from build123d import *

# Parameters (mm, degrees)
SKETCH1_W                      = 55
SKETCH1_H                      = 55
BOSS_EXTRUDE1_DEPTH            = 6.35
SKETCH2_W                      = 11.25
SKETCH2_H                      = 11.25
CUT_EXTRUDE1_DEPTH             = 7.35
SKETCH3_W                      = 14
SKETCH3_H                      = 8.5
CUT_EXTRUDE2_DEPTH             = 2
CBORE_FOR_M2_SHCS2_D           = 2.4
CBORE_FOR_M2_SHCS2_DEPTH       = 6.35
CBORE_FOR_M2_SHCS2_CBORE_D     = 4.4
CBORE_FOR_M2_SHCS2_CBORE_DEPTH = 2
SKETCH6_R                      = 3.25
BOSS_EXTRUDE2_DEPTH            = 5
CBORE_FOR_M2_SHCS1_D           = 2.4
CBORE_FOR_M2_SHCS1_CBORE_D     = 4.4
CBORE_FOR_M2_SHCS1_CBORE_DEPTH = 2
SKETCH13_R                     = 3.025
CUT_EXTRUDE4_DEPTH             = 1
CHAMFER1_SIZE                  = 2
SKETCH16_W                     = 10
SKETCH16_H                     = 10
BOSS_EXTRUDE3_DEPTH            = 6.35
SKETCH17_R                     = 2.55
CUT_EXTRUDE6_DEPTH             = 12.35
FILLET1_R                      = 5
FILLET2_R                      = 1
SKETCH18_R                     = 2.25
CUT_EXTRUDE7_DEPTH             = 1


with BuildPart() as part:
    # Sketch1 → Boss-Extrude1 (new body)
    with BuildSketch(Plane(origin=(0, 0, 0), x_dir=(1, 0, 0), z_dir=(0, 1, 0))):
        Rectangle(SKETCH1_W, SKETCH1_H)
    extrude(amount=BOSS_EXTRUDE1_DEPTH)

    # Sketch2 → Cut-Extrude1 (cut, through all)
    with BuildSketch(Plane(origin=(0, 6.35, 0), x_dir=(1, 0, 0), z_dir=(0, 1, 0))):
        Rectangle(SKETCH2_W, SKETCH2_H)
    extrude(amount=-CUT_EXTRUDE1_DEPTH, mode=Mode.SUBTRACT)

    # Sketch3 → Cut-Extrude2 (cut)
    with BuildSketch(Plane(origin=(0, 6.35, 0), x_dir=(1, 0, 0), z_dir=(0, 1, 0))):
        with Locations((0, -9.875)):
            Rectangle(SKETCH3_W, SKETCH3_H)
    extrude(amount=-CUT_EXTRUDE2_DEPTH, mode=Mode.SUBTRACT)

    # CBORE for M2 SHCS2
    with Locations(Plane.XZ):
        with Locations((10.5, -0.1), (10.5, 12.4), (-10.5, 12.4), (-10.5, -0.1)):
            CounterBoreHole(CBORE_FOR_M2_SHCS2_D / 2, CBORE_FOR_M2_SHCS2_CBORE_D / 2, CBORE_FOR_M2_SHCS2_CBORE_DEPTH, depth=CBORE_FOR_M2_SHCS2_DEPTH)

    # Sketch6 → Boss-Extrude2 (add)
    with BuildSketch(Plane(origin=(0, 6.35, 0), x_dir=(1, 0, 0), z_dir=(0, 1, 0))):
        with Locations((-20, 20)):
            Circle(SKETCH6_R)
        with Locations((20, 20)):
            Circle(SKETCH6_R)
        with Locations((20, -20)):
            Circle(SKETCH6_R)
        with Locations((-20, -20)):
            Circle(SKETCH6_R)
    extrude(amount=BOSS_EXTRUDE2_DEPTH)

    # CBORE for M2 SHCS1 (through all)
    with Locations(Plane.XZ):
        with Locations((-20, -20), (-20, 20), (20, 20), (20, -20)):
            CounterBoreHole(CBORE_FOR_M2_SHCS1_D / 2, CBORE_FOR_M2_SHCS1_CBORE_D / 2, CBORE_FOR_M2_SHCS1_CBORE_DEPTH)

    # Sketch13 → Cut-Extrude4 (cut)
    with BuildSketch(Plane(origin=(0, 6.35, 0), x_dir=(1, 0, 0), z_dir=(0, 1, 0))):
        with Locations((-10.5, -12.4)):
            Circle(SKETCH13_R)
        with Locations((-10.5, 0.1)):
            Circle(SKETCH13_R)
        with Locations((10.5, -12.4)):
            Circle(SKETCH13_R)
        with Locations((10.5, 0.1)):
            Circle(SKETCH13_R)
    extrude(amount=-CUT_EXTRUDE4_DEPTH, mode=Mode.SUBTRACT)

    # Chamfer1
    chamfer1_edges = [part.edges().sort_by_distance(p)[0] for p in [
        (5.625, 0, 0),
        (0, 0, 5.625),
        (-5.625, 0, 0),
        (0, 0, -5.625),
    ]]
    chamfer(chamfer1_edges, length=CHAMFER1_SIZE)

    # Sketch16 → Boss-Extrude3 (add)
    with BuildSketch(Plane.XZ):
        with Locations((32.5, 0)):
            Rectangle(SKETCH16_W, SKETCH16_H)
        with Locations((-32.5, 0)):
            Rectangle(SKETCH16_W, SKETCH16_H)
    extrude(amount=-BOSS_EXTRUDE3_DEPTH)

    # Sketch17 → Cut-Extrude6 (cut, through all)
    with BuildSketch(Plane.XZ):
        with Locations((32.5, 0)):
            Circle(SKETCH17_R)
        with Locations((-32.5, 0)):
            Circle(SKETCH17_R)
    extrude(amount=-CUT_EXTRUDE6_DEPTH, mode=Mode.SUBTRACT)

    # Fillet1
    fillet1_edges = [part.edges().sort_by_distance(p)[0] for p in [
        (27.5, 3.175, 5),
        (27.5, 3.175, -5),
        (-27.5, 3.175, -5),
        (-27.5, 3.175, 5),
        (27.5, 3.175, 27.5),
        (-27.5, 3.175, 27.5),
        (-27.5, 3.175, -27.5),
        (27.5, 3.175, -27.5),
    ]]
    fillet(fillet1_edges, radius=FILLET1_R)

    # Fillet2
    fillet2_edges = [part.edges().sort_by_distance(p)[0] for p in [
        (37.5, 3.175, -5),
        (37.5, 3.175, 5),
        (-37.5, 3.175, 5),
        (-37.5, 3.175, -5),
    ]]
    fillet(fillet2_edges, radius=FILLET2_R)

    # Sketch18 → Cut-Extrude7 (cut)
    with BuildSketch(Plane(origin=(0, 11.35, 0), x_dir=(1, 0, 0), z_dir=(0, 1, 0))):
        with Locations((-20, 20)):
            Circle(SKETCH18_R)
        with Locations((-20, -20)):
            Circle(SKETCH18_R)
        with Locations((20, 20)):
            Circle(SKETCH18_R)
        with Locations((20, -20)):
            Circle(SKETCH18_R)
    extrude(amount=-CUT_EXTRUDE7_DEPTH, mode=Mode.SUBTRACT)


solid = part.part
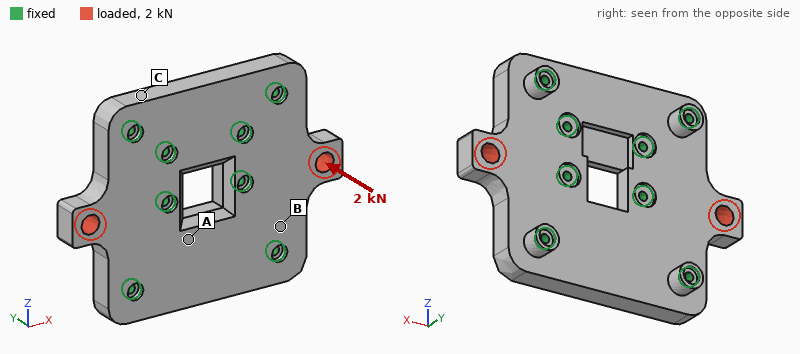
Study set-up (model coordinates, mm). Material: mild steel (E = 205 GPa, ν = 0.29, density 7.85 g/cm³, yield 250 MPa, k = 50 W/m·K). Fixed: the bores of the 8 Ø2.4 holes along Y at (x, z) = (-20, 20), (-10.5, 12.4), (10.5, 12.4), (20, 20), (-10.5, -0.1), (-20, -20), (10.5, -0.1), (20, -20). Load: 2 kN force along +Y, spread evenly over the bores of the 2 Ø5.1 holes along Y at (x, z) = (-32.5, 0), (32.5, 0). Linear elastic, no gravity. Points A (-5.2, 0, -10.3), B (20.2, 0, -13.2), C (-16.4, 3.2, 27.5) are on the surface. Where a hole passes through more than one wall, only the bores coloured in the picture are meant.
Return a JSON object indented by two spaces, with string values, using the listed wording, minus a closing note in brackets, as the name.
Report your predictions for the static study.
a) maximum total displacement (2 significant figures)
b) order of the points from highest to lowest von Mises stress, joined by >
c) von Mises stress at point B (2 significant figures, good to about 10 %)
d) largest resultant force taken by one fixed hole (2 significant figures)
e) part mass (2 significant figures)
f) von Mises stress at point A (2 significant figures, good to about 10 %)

{
  "maximum total displacement": "36 µm",
  "order of the points from highest to lowest von Mises stress, joined by >": "B > A > C",
  "von Mises stress at point B": "49 MPa",
  "largest resultant force taken by one fixed hole": "690 N",
  "part mass": "150 g",
  "von Mises stress at point A": "20 MPa"
}
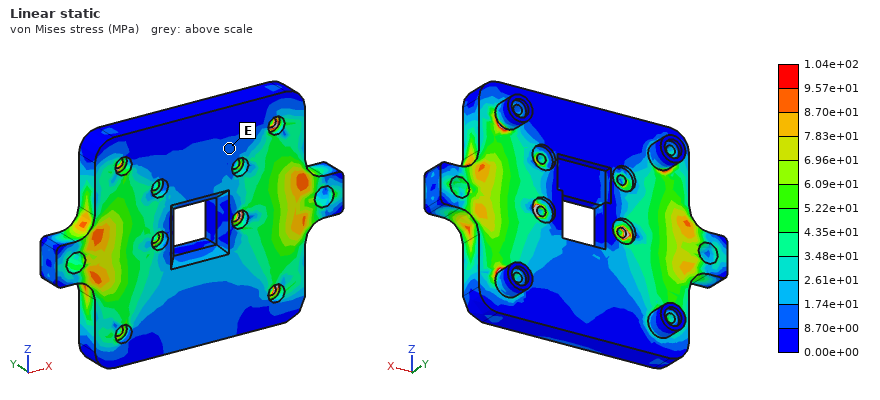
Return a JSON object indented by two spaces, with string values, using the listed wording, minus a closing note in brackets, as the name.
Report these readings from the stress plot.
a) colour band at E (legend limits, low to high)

{
  "colour band at E": "8.70e+00 to 1.74e+01 MPa"
}
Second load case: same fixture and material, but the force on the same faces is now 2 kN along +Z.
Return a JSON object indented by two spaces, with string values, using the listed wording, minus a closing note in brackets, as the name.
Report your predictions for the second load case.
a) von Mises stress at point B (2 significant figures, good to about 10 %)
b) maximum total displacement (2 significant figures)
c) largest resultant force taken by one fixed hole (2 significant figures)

{
  "von Mises stress at point B": "7.3 MPa",
  "maximum total displacement": "5.1 µm",
  "largest resultant force taken by one fixed hole": "440 N"
}
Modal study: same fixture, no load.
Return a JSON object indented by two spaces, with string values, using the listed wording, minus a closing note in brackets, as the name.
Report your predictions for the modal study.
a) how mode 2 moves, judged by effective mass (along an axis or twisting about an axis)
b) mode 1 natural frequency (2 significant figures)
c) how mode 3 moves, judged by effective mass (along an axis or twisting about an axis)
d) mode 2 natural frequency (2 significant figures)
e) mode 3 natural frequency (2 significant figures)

{
  "how mode 2 moves, judged by effective mass": "twisting about Z",
  "mode 1 natural frequency": "12 kHz",
  "how mode 3 moves, judged by effective mass": "along Y",
  "mode 2 natural frequency": "13 kHz",
  "mode 3 natural frequency": "18 kHz"
}
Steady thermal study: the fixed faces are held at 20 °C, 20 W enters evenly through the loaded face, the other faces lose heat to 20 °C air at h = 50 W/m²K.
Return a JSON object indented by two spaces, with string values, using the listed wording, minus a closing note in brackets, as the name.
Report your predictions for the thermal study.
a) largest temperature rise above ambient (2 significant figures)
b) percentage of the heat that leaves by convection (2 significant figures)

{
  "largest temperature rise above ambient": "41 K",
  "percentage of the heat that leaves by convection": "12 %"
}
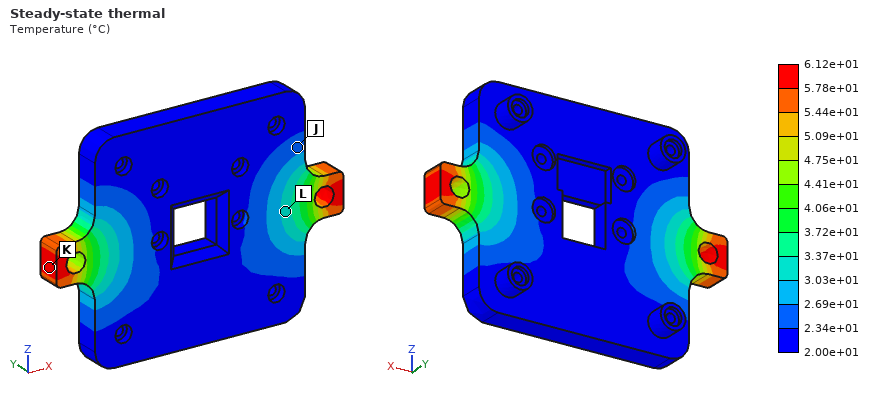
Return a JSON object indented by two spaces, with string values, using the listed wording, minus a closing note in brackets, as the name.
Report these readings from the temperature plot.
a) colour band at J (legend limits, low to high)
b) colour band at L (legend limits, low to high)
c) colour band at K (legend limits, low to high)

{
  "colour band at J": "2.34e+01 to 2.69e+01 °C",
  "colour band at L": "3.03e+01 to 3.37e+01 °C",
  "colour band at K": "5.78e+01 to 6.12e+01 °C"
}
